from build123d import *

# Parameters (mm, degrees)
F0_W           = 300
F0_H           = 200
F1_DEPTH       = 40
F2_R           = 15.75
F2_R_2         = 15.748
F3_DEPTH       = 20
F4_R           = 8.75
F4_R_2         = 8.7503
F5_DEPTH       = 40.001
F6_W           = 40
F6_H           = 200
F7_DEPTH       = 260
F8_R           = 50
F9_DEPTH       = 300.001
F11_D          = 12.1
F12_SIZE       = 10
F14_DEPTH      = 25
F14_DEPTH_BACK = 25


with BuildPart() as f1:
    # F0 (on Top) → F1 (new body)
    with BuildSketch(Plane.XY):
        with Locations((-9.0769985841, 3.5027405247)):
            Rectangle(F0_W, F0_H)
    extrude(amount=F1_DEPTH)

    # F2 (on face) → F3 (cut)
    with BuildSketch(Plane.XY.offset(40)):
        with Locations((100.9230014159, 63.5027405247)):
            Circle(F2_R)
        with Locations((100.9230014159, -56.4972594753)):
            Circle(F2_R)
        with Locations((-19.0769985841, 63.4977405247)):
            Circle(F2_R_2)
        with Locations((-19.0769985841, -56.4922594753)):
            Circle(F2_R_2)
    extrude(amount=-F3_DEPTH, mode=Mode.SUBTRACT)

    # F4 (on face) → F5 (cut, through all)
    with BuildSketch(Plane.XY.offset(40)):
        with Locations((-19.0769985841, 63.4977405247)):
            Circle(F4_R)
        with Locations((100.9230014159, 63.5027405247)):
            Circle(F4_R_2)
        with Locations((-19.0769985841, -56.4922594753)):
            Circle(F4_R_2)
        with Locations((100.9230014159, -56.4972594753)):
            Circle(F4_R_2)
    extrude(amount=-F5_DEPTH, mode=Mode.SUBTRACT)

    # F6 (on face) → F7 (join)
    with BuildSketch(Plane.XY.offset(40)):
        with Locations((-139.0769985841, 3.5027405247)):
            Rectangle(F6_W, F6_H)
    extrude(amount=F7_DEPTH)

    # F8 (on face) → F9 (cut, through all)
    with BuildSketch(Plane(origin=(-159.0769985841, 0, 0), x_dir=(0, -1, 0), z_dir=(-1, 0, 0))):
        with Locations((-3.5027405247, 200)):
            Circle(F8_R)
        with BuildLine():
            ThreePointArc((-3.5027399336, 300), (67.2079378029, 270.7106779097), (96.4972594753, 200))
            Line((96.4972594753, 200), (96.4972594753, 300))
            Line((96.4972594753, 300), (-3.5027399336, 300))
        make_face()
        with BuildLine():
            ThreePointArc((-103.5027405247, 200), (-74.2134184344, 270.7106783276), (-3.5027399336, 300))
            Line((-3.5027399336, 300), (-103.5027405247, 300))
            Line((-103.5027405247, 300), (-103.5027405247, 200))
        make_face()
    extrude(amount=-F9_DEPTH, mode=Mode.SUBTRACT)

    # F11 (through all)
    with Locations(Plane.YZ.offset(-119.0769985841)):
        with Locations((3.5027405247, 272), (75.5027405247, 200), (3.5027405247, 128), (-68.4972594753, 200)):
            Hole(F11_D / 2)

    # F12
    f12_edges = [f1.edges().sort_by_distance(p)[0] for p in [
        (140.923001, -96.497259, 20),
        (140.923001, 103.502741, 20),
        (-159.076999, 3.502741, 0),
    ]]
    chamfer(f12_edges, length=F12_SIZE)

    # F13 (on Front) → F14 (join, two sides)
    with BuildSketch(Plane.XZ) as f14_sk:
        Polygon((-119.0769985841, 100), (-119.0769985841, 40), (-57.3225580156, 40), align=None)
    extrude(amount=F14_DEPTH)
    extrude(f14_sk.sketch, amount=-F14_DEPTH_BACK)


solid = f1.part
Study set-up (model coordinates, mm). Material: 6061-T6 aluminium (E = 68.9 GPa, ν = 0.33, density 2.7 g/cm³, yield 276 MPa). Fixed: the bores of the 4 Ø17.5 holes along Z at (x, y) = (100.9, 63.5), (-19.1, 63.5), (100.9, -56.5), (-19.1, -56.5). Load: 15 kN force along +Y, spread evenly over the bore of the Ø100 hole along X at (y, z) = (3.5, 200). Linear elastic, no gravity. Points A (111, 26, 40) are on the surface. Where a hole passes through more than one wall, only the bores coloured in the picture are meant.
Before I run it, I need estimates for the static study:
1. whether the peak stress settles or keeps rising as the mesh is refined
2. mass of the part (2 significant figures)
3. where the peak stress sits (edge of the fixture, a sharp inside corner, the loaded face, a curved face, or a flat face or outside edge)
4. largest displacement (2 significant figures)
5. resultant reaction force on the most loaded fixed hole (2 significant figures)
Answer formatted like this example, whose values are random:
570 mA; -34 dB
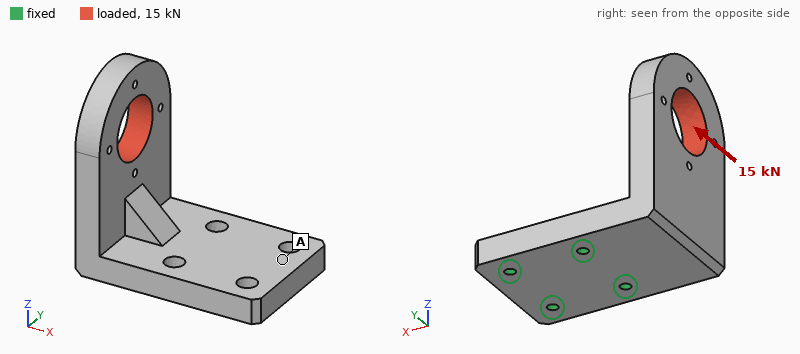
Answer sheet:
keeps rising; 11 kg; edge of the fixture; 0.52 mm; 29 kN
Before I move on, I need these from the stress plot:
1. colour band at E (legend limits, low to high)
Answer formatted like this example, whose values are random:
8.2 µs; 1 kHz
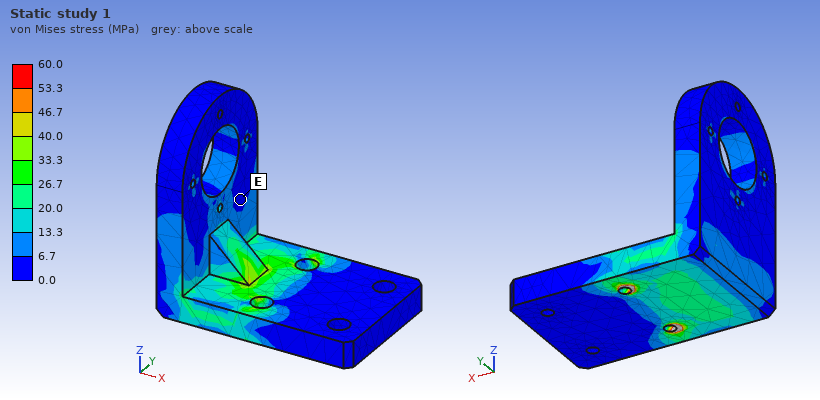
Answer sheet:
0.0 to 6.7 MPa
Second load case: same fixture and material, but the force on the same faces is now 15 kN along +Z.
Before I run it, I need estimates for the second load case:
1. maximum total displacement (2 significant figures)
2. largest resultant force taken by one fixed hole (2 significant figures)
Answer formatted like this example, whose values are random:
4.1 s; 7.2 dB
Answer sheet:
0.59 mm; 16 kN
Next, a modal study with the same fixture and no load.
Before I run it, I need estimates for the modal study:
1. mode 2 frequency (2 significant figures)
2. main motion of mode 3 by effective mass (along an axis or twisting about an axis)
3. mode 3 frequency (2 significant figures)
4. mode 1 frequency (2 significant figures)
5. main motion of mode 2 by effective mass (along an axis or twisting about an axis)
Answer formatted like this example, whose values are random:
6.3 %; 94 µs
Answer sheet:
570 Hz; along Z; 980 Hz; 320 Hz; along Y
